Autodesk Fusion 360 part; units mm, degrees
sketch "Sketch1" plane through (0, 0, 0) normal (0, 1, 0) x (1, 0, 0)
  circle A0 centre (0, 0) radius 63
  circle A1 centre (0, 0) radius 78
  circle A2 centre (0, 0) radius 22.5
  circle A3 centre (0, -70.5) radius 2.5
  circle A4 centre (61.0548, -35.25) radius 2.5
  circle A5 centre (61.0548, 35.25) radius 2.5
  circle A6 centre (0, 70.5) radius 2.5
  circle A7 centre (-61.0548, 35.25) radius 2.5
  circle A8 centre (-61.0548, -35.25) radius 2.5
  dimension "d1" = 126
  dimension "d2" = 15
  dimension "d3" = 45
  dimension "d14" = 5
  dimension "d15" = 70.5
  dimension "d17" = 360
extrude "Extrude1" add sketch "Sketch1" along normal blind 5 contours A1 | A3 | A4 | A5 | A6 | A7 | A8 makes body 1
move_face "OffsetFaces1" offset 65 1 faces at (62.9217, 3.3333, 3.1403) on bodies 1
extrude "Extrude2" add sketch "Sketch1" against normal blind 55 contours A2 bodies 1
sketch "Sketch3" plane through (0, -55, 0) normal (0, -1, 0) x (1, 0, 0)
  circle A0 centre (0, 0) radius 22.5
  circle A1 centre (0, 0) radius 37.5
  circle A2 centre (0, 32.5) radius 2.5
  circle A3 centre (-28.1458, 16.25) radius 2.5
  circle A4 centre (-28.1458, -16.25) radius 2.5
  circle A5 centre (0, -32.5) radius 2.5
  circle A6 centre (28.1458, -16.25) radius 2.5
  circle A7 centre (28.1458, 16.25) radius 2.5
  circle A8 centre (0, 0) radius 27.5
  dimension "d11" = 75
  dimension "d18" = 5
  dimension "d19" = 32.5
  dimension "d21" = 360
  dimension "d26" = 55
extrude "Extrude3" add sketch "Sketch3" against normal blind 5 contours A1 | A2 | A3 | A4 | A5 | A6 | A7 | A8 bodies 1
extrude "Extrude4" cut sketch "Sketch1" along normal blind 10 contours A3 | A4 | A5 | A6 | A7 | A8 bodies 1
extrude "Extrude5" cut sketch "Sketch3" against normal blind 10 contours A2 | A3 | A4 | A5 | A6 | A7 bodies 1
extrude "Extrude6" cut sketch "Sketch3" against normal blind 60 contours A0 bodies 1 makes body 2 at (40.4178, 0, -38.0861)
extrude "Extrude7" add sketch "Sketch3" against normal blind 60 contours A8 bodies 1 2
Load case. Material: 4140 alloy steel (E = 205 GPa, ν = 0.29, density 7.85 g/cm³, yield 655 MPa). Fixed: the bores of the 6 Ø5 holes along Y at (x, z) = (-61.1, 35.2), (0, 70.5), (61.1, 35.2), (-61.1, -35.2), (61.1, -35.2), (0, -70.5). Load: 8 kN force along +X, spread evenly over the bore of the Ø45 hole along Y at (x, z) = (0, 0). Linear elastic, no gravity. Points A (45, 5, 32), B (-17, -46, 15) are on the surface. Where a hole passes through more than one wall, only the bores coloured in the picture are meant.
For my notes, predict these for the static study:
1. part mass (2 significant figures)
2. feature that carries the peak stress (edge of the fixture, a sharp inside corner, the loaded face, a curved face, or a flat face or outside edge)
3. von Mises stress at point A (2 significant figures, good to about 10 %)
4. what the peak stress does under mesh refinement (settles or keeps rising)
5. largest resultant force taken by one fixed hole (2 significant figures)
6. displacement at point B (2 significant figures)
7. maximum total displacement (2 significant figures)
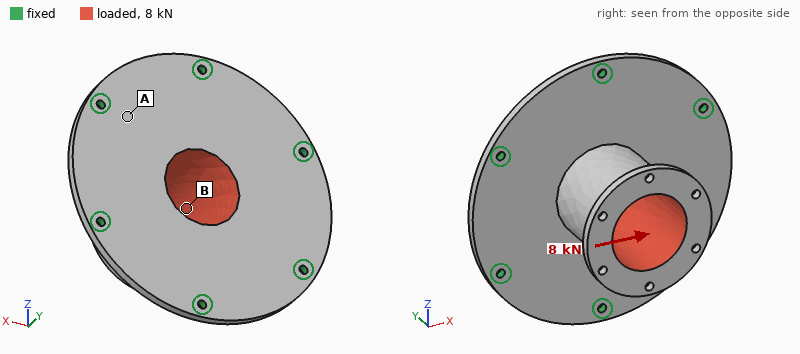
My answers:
1.1 kg
edge of the fixture
38 MPa
keeps rising
2.1 kN
0.15 mm
0.20 mm
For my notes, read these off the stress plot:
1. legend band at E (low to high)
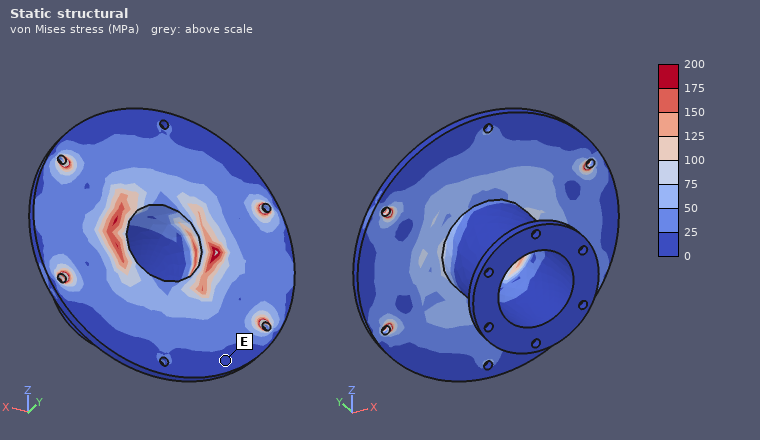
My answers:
0 to 25 MPa
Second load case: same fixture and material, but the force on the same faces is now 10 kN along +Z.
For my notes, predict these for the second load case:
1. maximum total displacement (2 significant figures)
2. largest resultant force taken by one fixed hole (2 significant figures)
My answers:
0.25 mm
3.0 kN
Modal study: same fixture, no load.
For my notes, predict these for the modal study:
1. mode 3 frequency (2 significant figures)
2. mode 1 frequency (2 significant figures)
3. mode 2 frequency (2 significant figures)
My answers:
1500 Hz
1500 Hz
1500 Hz
